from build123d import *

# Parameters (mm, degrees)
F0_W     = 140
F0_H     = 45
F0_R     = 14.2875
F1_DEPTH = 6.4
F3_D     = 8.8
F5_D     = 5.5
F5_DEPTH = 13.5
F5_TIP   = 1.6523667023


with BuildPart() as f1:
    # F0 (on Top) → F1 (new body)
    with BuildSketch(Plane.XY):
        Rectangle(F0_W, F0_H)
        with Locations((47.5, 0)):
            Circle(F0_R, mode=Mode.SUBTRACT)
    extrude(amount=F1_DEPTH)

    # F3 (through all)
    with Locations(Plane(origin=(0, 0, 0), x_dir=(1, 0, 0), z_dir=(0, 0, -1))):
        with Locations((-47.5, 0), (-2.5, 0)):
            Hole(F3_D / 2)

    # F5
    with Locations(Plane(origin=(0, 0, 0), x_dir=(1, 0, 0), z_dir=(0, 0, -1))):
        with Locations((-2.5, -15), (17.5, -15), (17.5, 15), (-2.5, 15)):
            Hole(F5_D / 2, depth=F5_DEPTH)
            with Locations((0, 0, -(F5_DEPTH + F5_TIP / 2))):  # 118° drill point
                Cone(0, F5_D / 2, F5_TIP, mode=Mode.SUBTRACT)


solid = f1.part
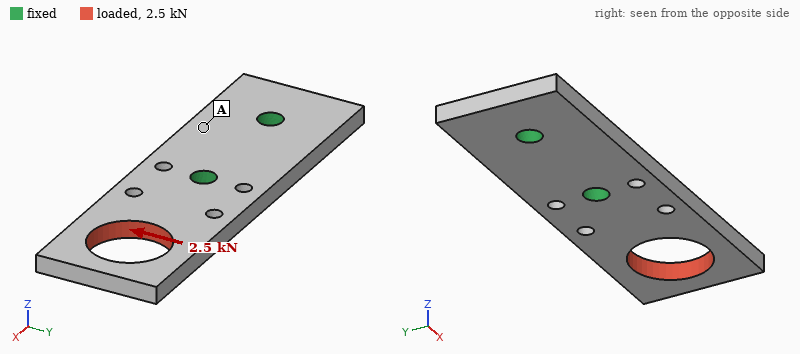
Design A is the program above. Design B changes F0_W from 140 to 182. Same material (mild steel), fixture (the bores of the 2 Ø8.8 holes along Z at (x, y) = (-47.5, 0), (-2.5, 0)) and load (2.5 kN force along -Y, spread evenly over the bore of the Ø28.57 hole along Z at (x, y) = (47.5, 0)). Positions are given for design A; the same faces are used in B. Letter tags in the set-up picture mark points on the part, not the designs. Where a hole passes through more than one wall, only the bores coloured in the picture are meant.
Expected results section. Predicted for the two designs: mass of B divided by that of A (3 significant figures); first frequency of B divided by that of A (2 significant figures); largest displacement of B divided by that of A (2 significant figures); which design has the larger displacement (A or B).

1.35
0.51
1.2
B
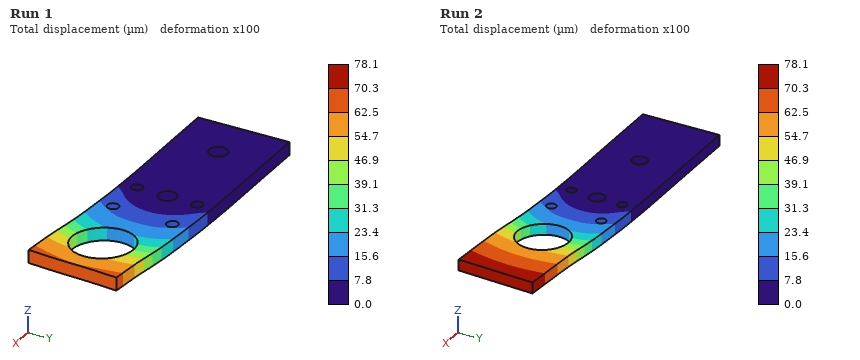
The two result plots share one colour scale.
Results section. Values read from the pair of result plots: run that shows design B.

Run 2
